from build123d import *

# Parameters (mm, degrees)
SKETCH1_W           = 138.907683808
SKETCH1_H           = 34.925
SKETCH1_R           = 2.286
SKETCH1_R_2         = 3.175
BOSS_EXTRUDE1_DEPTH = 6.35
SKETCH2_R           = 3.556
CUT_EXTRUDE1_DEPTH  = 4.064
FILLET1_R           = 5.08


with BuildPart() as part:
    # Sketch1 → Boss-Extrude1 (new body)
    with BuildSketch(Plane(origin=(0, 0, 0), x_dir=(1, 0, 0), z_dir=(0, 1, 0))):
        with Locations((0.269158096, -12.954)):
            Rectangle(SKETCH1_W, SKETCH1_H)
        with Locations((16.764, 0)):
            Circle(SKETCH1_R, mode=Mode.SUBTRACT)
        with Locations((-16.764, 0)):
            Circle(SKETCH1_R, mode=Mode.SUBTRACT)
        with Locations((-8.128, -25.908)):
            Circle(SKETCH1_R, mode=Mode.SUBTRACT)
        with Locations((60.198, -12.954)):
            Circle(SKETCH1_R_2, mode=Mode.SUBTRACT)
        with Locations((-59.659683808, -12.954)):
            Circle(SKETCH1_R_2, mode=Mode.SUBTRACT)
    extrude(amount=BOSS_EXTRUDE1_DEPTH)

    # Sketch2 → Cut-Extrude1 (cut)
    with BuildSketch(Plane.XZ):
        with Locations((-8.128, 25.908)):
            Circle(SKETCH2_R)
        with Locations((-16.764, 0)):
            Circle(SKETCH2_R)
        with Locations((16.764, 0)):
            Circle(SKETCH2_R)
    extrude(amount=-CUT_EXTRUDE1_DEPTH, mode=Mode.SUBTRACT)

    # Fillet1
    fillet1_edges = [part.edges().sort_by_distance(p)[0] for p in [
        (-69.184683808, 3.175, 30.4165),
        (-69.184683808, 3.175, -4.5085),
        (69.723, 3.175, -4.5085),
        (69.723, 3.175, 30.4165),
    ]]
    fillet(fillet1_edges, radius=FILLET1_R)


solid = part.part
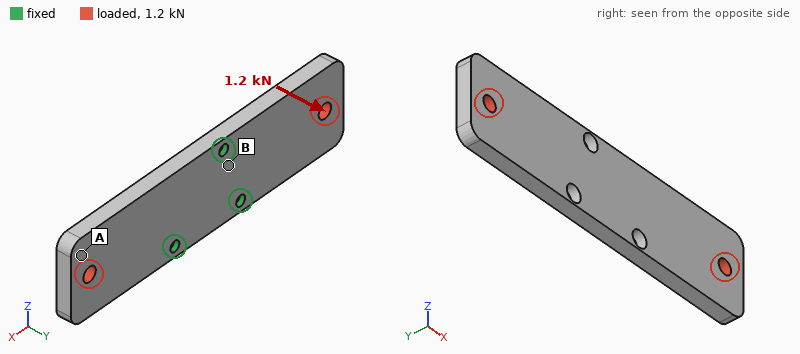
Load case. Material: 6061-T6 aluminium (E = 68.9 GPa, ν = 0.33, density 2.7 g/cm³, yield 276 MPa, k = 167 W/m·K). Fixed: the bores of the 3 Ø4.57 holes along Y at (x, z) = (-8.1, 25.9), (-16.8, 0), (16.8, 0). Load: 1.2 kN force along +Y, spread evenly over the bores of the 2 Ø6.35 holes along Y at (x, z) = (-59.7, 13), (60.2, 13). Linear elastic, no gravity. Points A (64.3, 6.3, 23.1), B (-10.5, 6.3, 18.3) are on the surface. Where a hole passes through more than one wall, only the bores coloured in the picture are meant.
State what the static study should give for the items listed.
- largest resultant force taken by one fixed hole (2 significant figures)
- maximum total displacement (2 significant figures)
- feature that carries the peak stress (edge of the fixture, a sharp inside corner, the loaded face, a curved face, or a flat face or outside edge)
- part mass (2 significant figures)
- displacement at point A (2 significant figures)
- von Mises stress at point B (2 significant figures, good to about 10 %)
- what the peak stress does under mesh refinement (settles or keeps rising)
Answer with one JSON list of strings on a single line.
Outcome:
["2.1 kN", "0.81 mm", "edge of the fixture", "80 g", "0.71 mm", "79 MPa", "keeps rising"]
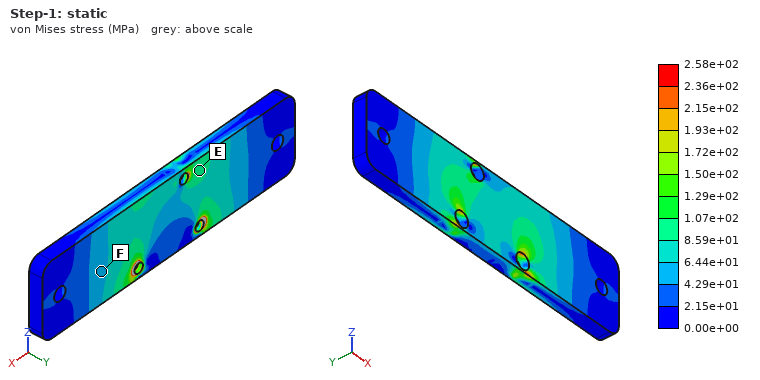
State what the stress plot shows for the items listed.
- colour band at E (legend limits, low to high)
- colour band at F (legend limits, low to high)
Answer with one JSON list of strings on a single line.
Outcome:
["8.59e+01 to 1.07e+02 MPa", "4.29e+01 to 6.44e+01 MPa"]
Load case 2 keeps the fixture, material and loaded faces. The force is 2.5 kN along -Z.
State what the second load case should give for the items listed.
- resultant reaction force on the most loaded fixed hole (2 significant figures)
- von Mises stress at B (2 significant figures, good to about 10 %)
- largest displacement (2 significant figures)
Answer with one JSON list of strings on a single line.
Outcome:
["2.0 kN", "19 MPa", "0.10 mm"]
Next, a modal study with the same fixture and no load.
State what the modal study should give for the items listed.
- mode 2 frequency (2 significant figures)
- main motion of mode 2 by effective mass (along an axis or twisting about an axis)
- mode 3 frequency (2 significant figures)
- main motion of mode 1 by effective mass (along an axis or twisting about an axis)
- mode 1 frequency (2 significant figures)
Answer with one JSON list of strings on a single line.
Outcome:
["1400 Hz", "along Y", "4200 Hz", "along Y", "1300 Hz"]
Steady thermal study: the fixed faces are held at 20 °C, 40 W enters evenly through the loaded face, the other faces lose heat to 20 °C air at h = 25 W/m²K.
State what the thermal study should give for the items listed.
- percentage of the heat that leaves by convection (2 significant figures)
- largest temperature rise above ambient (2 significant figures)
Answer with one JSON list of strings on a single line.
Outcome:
["11 %", "32 K"]
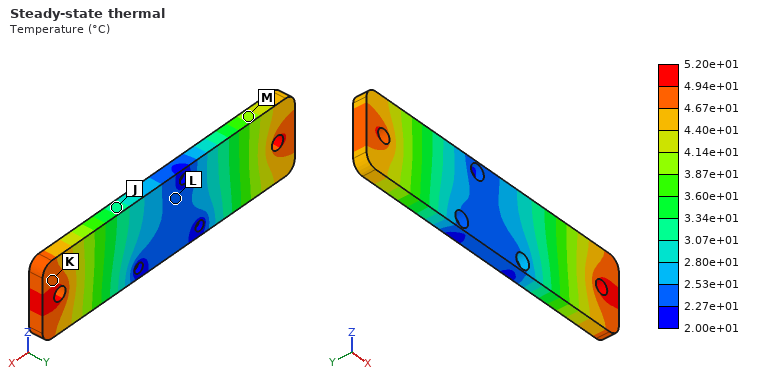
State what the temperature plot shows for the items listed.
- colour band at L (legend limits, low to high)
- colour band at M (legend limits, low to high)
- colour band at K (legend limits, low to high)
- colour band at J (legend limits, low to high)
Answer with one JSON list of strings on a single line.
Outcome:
["2.27e+01 to 2.53e+01 °C", "3.87e+01 to 4.14e+01 °C", "4.67e+01 to 4.94e+01 °C", "3.07e+01 to 3.34e+01 °C"]
